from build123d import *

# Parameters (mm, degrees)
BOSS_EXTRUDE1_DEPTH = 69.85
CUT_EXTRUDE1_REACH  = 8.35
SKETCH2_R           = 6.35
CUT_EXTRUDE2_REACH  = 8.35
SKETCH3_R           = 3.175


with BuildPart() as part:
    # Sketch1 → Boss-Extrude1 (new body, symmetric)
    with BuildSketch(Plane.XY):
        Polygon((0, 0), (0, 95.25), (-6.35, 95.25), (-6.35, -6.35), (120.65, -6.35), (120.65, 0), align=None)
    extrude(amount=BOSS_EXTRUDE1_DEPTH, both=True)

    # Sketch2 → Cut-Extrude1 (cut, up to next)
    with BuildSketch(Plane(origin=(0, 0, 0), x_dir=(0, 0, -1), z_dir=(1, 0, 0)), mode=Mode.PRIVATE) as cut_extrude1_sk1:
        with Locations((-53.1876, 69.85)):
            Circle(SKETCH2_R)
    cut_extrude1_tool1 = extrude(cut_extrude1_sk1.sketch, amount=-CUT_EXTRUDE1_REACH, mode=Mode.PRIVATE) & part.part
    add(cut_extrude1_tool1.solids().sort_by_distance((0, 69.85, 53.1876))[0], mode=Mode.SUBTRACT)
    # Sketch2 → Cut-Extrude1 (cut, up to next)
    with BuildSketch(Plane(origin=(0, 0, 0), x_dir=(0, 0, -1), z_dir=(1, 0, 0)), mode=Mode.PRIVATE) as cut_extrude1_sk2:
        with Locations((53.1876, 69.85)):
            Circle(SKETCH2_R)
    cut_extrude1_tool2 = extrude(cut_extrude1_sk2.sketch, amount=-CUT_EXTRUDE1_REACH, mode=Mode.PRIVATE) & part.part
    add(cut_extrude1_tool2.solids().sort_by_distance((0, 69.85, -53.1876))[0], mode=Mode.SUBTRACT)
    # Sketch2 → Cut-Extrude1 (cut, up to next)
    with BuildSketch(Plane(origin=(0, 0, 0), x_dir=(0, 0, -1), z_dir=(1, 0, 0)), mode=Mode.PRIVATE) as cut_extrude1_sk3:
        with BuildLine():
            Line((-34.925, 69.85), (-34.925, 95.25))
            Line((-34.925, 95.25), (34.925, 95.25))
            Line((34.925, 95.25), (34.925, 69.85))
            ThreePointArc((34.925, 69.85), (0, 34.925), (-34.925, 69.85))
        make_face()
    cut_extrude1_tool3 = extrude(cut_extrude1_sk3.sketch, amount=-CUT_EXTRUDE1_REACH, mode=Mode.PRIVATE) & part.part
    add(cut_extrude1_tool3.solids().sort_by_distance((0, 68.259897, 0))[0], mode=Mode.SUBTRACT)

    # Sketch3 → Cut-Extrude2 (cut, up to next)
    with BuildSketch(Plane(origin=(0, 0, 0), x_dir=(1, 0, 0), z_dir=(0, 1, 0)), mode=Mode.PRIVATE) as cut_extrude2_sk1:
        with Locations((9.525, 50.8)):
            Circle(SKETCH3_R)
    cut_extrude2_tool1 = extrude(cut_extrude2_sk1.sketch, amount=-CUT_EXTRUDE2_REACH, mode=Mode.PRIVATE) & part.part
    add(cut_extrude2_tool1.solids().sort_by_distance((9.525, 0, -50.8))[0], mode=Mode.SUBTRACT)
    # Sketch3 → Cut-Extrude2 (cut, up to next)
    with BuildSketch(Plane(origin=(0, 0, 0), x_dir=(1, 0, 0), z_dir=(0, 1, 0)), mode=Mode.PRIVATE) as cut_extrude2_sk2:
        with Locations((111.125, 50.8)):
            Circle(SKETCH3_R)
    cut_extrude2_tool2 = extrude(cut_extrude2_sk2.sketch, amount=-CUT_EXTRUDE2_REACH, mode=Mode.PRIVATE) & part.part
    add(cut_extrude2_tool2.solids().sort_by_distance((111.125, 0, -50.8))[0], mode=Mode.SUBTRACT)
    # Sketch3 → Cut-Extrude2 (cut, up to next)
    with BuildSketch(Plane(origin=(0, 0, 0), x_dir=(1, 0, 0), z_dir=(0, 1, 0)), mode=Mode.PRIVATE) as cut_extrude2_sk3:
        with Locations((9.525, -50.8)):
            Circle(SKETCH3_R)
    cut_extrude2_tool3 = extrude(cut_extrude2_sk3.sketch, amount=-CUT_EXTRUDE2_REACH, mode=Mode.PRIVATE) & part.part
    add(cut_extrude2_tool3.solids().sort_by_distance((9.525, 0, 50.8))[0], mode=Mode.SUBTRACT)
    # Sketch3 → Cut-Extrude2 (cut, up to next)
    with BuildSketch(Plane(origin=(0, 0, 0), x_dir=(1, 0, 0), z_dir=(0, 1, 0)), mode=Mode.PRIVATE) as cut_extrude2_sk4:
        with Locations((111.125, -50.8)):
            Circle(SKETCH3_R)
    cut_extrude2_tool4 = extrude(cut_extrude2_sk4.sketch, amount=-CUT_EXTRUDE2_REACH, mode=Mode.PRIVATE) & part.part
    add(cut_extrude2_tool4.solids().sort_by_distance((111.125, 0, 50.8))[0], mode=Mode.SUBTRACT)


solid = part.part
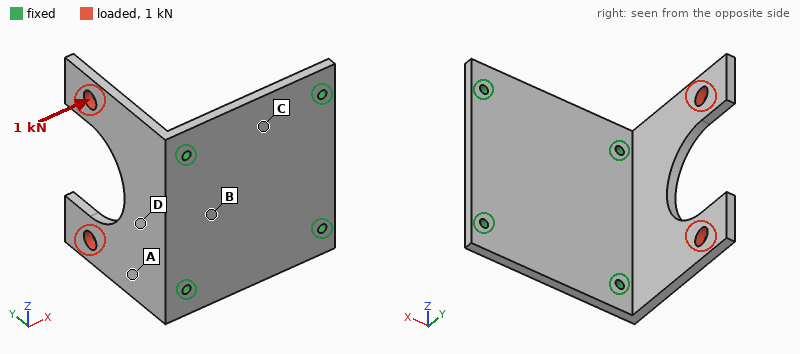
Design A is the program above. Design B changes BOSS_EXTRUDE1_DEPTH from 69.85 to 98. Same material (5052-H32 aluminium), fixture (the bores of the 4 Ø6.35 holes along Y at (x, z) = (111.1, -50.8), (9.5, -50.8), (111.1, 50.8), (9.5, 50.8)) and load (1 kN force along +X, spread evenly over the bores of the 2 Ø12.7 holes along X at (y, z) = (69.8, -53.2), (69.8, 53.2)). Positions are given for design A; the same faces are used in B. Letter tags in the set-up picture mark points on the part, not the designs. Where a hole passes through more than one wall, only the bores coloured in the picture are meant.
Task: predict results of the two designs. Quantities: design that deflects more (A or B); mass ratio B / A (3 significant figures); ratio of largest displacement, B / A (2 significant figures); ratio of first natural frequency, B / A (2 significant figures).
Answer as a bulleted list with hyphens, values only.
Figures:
- A
- 1.46
- 0.68
- 0.87
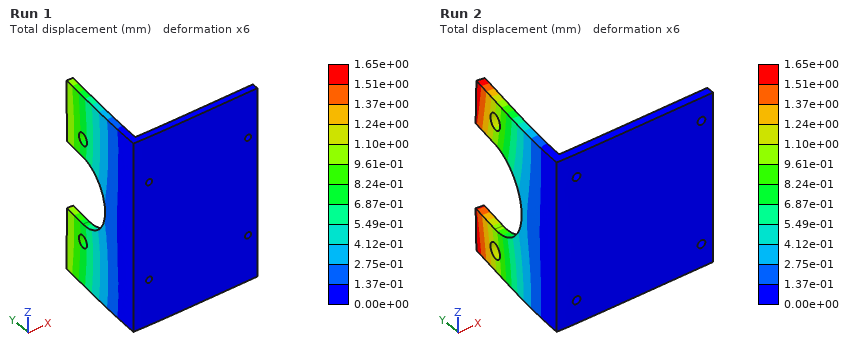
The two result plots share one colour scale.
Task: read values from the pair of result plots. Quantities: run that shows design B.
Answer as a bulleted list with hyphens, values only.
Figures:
- Run 1
